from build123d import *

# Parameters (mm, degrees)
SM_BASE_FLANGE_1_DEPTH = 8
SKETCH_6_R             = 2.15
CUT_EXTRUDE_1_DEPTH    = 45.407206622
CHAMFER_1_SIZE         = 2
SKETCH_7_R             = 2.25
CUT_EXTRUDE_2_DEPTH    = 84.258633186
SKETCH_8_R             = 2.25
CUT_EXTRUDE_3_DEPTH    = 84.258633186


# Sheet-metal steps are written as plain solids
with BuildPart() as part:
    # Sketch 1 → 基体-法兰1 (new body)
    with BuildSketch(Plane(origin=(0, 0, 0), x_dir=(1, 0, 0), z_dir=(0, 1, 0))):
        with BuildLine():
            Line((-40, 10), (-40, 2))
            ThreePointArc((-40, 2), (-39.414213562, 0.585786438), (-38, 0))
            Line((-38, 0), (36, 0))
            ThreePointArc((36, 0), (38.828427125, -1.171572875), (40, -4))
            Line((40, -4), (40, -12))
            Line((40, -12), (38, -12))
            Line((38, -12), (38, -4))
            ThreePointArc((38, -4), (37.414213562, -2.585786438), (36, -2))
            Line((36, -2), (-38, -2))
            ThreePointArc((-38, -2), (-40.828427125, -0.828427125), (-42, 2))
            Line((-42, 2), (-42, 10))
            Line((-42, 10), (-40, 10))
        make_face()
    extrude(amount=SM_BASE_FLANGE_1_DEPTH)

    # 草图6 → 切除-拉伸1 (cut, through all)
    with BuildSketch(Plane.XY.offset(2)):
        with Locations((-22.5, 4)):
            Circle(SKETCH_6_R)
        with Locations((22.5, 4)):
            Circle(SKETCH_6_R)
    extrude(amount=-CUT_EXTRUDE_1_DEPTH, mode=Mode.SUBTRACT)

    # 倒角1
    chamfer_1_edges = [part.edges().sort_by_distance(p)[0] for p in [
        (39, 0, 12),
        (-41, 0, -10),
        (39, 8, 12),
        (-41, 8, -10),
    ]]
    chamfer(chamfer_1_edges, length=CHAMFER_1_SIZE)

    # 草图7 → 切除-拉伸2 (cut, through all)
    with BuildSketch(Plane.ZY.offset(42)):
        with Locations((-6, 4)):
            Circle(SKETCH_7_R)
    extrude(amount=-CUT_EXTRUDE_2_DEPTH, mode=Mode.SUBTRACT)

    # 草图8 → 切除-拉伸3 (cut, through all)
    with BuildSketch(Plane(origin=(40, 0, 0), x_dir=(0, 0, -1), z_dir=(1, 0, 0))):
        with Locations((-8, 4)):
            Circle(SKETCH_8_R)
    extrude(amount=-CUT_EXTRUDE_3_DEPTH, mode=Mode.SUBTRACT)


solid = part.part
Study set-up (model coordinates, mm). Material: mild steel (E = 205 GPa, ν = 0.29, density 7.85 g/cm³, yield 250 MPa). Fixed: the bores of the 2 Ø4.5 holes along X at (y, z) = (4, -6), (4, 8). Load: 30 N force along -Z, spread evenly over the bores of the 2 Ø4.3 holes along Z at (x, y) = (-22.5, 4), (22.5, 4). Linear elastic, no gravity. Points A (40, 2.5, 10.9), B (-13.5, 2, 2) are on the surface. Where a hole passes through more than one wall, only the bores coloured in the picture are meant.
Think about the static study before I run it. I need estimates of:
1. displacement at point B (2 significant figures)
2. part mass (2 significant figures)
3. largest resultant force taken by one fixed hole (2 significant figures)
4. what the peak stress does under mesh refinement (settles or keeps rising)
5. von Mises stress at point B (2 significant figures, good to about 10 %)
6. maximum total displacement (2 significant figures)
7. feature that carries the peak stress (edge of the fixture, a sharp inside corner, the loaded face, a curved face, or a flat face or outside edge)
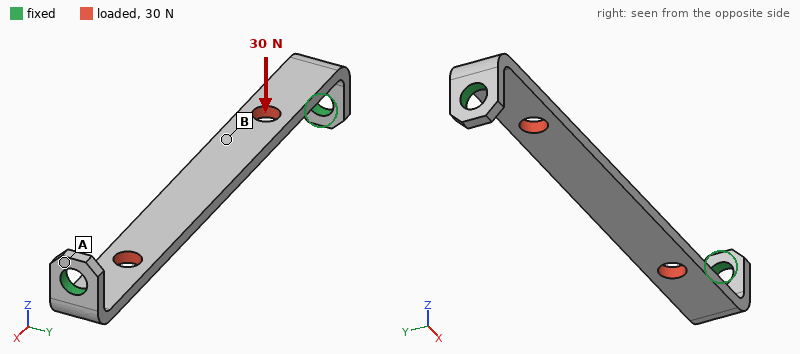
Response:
38 µm
11 g
15 N
keeps rising
14 MPa
43 µm
edge of the fixture
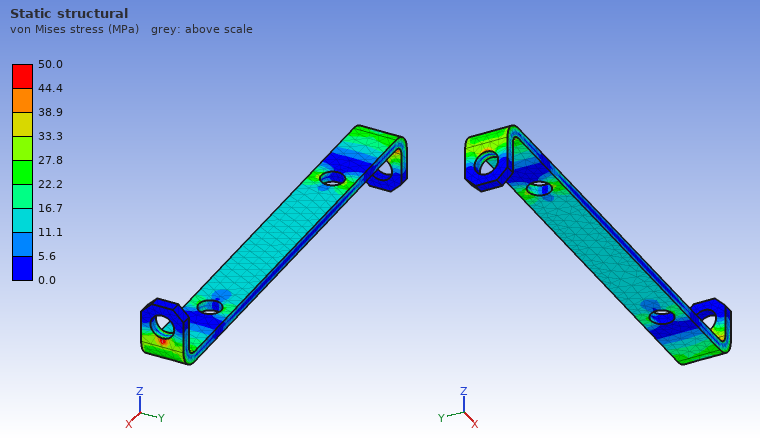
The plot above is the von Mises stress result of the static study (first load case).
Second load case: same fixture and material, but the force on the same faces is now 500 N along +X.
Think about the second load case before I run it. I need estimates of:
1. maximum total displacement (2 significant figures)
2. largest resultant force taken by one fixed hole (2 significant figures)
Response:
62 µm
250 N
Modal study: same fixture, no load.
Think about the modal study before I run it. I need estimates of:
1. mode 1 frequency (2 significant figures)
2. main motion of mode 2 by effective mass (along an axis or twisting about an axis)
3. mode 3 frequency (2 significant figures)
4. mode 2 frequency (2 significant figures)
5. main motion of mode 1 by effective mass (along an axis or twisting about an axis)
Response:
1400 Hz
along Y
4300 Hz
3700 Hz
along Z
